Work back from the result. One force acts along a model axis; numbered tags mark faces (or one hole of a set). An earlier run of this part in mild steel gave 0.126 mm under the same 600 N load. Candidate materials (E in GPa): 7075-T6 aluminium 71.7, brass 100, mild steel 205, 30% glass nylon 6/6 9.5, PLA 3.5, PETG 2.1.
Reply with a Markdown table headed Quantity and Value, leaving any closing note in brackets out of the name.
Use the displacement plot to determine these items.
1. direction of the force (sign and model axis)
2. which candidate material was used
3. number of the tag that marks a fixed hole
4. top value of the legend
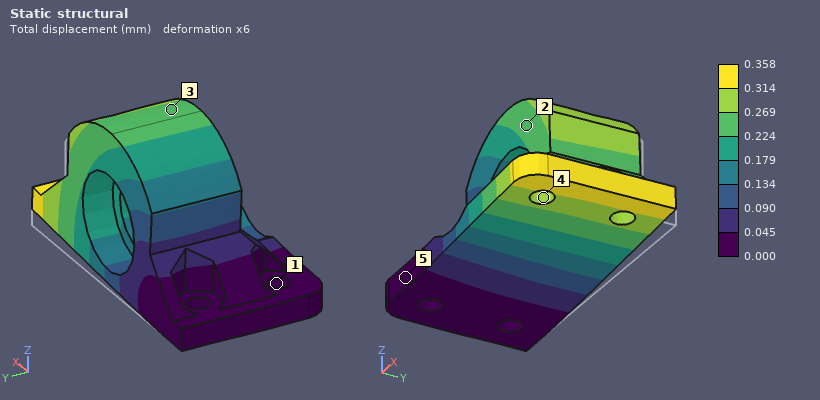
| Quantity | Value |
|---|---|
| direction of the force | +Z |
| which candidate material was used | 7075-T6 aluminium |
| number of the tag that marks a fixed hole | 1 |
| top value of the legend | 0.358 mm |
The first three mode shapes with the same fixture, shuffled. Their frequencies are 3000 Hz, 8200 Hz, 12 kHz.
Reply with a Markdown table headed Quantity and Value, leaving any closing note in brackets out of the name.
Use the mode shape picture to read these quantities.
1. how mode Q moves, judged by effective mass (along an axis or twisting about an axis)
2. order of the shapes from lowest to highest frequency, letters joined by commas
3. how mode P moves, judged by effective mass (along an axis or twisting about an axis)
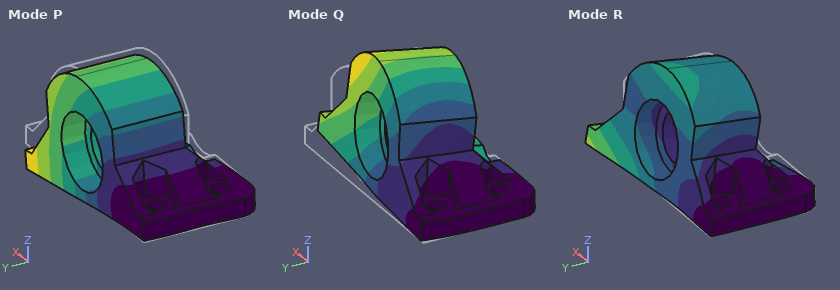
| Quantity | Value |
|---|---|
| how mode Q moves, judged by effective mass | along Y |
| order of the shapes from lowest to highest frequency, letters joined by commas | P, Q, R |
| how mode P moves, judged by effective mass | along Z |
